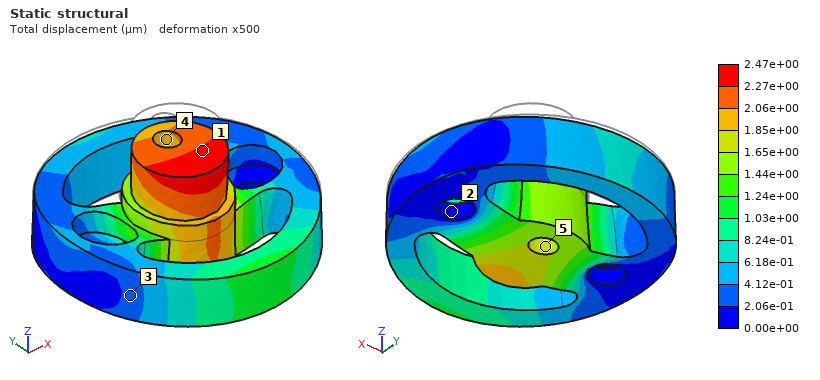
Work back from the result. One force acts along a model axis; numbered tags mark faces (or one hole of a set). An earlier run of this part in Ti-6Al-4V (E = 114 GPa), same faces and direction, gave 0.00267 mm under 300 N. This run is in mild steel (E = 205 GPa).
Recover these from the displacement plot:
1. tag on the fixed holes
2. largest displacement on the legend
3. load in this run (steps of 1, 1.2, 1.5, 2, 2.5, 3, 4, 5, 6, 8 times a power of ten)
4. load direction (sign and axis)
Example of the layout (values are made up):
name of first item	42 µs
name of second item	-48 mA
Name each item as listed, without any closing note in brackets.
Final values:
tag on the fixed holes	2
largest displacement on the legend	2.47e+00 µm
load in this run	500 N
load direction	-Z
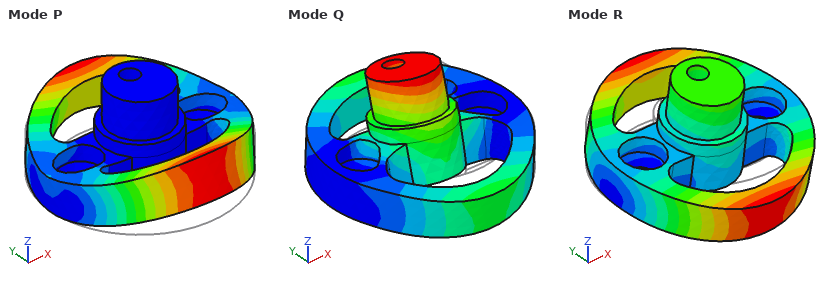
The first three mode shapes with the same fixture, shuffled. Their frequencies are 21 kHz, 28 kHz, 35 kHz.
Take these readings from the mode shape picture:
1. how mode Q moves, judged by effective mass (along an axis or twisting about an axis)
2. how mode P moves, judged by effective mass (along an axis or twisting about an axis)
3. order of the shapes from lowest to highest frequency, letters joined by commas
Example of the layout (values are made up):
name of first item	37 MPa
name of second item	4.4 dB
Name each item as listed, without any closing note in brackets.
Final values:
how mode Q moves, judged by effective mass	along Y
how mode P moves, judged by effective mass	along Z
order of the shapes from lowest to highest frequency, letters joined by commas	R, P, Q
